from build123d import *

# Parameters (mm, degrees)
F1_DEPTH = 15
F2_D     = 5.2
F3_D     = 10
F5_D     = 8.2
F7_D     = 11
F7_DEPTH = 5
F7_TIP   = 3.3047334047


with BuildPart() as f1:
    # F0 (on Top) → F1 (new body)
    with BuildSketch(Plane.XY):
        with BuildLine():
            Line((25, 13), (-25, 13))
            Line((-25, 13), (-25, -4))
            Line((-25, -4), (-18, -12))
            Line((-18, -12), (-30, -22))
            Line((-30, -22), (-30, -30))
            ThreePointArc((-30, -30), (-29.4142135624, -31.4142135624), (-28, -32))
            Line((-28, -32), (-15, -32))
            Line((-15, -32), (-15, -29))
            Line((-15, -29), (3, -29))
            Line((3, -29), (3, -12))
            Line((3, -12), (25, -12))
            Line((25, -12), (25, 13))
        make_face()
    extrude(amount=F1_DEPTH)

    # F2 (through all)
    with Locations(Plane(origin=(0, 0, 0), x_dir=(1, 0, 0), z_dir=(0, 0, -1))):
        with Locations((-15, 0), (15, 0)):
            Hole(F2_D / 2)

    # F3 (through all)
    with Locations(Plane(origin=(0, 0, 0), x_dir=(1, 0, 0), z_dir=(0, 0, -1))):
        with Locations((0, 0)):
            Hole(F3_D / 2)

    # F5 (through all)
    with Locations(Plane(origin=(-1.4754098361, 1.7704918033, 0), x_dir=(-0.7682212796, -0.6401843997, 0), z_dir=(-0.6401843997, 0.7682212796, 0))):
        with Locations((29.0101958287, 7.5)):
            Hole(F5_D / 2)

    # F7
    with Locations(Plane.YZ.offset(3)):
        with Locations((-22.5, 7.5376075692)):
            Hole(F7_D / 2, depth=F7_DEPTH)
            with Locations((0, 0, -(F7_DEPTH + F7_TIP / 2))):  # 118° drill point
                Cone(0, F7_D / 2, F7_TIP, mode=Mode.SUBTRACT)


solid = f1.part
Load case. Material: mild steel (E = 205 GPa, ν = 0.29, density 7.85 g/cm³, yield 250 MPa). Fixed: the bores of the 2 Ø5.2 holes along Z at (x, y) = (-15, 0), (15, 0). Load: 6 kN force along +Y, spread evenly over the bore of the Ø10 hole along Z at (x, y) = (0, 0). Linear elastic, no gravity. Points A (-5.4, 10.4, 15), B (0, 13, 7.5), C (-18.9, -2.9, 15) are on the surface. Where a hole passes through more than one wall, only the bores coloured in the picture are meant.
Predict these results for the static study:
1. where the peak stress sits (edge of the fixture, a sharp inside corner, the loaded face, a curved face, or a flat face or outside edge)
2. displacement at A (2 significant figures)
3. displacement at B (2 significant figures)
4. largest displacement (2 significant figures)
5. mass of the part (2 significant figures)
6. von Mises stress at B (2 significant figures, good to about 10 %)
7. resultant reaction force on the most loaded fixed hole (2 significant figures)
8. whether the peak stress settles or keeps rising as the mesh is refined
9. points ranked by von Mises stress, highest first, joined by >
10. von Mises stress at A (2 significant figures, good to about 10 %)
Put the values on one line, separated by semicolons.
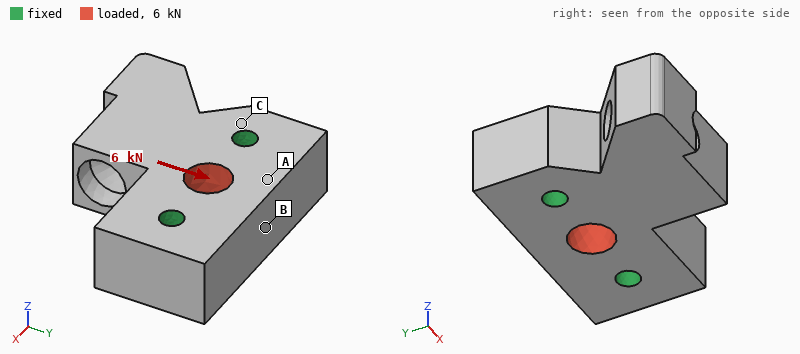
edge of the fixture; 1.4 µm; 1.6 µm; 2.5 µm; 180 g; 23 MPa; 3.0 kN; keeps rising; B > A > C; 14 MPa
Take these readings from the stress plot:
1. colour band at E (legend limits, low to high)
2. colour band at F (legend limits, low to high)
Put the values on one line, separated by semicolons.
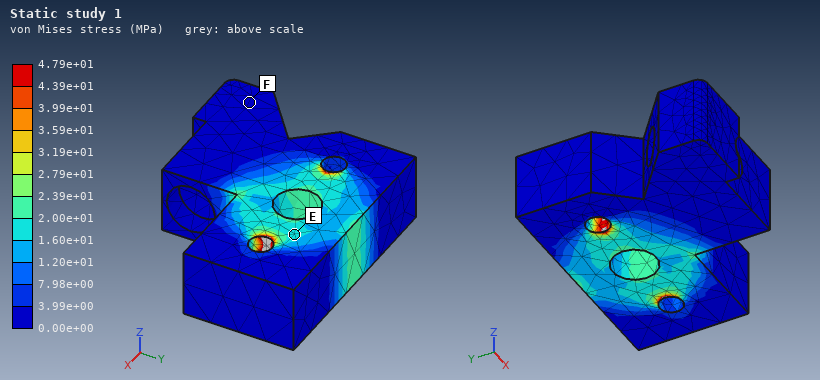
1.60e+01 to 2.00e+01 MPa; 0.00e+00 to 3.99e+00 MPa
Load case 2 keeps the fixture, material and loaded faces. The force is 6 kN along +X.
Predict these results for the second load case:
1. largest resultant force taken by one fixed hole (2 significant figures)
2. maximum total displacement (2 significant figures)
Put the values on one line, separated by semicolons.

3.0 kN; 0.94 µm
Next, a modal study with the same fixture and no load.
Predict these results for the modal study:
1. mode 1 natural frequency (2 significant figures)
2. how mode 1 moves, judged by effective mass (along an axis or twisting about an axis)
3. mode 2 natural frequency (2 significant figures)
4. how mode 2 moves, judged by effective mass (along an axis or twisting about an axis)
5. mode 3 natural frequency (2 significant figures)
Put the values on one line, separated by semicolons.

9400 Hz; along Z; 14 kHz; along X; 18 kHz
